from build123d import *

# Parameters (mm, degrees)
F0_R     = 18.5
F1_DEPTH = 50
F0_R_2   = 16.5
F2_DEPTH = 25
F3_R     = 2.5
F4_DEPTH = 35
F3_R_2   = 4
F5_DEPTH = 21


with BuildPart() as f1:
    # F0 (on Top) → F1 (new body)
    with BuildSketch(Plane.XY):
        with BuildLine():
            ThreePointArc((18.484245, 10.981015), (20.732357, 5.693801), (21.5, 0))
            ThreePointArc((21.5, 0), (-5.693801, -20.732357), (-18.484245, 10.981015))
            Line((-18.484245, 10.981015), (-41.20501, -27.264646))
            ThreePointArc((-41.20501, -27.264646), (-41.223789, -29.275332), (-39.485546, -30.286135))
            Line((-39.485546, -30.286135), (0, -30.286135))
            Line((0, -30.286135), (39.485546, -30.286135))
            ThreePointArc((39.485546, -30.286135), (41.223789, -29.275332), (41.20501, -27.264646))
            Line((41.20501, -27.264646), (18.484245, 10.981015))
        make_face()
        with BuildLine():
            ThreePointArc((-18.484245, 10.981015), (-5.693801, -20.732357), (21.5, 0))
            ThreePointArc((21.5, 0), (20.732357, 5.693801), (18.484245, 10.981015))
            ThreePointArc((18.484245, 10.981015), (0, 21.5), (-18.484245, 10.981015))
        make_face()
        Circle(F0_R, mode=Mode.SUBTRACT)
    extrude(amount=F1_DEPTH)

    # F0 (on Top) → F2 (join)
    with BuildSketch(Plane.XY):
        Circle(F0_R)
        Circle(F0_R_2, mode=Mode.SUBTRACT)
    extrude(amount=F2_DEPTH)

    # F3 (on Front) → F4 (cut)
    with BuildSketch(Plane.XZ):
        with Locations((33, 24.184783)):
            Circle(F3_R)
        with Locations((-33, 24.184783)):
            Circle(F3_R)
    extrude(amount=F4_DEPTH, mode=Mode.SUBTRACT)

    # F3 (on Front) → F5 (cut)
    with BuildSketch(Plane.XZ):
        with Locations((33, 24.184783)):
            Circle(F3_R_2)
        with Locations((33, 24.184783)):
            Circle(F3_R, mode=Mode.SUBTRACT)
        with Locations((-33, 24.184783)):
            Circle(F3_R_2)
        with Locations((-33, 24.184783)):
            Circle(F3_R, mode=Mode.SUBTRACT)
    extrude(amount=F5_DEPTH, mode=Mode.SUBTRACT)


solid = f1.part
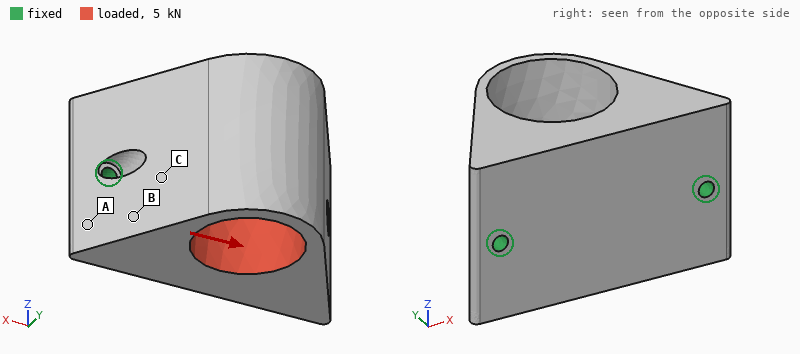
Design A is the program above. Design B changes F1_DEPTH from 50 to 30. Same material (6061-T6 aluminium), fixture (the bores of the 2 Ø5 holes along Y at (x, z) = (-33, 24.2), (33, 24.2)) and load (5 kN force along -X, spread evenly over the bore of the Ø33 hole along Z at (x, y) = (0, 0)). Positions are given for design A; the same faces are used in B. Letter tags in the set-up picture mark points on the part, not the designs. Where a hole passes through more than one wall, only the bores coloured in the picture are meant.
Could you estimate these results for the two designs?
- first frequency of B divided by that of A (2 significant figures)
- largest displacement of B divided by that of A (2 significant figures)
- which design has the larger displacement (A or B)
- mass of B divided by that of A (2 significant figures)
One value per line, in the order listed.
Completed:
1.1
1.3
B
0.62
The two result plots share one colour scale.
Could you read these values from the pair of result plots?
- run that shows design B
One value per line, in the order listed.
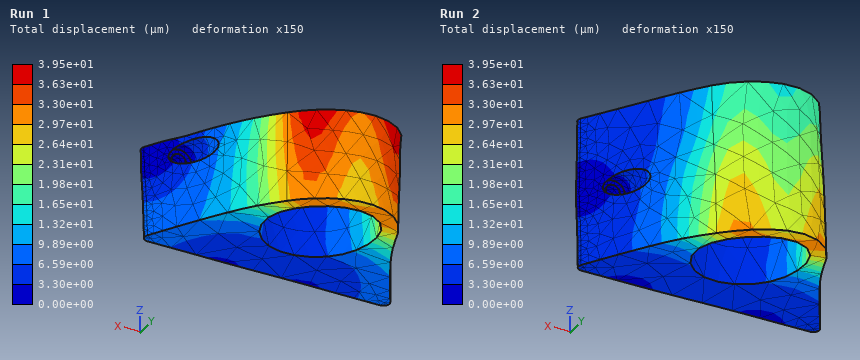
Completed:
Run 1
